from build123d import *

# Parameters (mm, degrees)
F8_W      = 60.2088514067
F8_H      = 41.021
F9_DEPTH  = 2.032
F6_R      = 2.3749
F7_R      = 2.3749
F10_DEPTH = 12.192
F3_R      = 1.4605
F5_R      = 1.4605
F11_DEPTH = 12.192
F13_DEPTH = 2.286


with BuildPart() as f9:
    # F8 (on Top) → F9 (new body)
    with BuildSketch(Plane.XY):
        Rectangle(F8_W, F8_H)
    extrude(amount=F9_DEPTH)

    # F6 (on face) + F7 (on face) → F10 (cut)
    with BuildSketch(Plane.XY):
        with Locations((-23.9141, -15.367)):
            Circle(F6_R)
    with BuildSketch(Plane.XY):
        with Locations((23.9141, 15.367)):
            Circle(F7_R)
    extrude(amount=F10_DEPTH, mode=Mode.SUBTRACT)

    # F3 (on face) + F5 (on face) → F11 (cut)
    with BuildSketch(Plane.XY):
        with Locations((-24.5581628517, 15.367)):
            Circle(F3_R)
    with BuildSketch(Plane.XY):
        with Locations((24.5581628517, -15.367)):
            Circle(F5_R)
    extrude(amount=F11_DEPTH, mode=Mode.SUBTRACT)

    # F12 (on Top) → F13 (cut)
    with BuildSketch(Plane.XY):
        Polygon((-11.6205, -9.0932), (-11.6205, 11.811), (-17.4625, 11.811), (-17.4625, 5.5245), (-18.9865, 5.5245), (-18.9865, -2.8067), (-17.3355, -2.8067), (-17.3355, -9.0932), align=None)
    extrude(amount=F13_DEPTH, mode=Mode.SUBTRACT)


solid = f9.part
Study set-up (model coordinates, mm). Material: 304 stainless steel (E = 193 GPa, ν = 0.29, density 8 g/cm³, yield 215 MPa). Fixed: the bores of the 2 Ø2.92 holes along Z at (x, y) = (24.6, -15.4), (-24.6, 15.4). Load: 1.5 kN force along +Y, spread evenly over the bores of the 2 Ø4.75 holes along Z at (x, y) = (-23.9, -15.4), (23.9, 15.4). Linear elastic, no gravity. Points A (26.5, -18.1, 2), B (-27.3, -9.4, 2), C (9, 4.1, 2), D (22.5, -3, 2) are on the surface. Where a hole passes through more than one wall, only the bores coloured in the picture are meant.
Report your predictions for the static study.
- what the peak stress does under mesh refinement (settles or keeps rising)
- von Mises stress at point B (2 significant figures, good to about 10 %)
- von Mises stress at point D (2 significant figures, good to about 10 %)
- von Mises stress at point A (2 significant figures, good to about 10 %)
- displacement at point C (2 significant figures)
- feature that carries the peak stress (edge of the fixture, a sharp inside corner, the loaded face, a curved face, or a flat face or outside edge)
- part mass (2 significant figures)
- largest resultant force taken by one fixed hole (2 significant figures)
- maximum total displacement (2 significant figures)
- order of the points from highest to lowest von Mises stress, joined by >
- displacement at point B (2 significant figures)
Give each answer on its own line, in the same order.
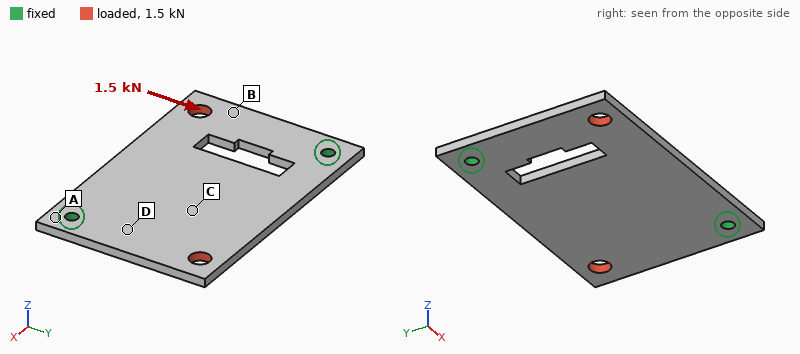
keeps rising
33 MPa
24 MPa
17 MPa
2.9 µm
edge of the fixture
37 g
770 N
6.5 µm
B > D > A > C
4.2 µm
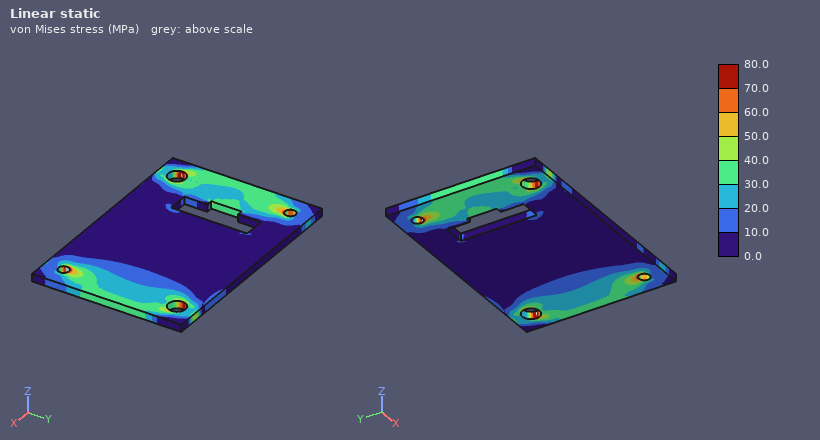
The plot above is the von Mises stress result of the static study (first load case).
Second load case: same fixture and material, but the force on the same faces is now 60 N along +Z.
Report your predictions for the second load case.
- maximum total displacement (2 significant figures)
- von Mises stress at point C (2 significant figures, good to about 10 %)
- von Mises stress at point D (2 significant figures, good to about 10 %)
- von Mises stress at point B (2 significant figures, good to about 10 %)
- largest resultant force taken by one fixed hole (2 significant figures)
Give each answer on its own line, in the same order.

68 µm
19 MPa
17 MPa
13 MPa
31 N
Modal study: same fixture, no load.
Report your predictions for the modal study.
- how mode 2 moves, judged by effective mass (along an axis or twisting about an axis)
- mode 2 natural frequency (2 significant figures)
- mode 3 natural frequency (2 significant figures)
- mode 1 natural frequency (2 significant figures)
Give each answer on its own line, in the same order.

along Z
1800 Hz
3700 Hz
1400 Hz
